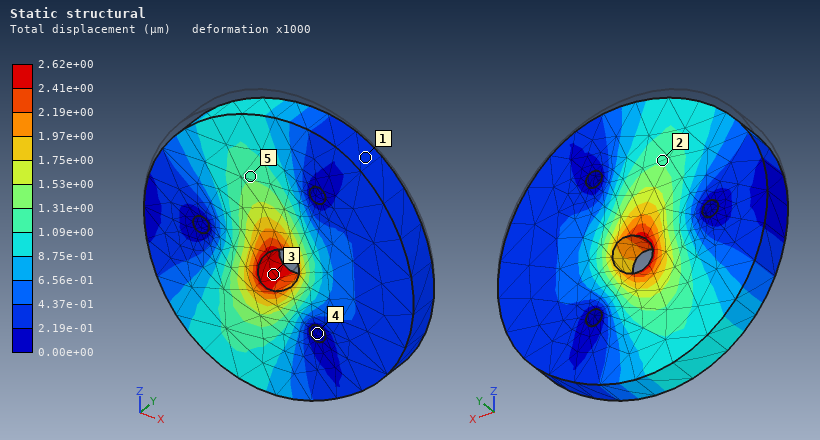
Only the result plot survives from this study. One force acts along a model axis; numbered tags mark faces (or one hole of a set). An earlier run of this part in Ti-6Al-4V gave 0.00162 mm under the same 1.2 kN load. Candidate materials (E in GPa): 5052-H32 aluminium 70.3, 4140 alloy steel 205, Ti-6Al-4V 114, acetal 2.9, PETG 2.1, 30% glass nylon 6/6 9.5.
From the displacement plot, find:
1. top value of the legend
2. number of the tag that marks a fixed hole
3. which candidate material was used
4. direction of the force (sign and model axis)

2.62e+00 µm
4
5052-H32 aluminium
-Z
